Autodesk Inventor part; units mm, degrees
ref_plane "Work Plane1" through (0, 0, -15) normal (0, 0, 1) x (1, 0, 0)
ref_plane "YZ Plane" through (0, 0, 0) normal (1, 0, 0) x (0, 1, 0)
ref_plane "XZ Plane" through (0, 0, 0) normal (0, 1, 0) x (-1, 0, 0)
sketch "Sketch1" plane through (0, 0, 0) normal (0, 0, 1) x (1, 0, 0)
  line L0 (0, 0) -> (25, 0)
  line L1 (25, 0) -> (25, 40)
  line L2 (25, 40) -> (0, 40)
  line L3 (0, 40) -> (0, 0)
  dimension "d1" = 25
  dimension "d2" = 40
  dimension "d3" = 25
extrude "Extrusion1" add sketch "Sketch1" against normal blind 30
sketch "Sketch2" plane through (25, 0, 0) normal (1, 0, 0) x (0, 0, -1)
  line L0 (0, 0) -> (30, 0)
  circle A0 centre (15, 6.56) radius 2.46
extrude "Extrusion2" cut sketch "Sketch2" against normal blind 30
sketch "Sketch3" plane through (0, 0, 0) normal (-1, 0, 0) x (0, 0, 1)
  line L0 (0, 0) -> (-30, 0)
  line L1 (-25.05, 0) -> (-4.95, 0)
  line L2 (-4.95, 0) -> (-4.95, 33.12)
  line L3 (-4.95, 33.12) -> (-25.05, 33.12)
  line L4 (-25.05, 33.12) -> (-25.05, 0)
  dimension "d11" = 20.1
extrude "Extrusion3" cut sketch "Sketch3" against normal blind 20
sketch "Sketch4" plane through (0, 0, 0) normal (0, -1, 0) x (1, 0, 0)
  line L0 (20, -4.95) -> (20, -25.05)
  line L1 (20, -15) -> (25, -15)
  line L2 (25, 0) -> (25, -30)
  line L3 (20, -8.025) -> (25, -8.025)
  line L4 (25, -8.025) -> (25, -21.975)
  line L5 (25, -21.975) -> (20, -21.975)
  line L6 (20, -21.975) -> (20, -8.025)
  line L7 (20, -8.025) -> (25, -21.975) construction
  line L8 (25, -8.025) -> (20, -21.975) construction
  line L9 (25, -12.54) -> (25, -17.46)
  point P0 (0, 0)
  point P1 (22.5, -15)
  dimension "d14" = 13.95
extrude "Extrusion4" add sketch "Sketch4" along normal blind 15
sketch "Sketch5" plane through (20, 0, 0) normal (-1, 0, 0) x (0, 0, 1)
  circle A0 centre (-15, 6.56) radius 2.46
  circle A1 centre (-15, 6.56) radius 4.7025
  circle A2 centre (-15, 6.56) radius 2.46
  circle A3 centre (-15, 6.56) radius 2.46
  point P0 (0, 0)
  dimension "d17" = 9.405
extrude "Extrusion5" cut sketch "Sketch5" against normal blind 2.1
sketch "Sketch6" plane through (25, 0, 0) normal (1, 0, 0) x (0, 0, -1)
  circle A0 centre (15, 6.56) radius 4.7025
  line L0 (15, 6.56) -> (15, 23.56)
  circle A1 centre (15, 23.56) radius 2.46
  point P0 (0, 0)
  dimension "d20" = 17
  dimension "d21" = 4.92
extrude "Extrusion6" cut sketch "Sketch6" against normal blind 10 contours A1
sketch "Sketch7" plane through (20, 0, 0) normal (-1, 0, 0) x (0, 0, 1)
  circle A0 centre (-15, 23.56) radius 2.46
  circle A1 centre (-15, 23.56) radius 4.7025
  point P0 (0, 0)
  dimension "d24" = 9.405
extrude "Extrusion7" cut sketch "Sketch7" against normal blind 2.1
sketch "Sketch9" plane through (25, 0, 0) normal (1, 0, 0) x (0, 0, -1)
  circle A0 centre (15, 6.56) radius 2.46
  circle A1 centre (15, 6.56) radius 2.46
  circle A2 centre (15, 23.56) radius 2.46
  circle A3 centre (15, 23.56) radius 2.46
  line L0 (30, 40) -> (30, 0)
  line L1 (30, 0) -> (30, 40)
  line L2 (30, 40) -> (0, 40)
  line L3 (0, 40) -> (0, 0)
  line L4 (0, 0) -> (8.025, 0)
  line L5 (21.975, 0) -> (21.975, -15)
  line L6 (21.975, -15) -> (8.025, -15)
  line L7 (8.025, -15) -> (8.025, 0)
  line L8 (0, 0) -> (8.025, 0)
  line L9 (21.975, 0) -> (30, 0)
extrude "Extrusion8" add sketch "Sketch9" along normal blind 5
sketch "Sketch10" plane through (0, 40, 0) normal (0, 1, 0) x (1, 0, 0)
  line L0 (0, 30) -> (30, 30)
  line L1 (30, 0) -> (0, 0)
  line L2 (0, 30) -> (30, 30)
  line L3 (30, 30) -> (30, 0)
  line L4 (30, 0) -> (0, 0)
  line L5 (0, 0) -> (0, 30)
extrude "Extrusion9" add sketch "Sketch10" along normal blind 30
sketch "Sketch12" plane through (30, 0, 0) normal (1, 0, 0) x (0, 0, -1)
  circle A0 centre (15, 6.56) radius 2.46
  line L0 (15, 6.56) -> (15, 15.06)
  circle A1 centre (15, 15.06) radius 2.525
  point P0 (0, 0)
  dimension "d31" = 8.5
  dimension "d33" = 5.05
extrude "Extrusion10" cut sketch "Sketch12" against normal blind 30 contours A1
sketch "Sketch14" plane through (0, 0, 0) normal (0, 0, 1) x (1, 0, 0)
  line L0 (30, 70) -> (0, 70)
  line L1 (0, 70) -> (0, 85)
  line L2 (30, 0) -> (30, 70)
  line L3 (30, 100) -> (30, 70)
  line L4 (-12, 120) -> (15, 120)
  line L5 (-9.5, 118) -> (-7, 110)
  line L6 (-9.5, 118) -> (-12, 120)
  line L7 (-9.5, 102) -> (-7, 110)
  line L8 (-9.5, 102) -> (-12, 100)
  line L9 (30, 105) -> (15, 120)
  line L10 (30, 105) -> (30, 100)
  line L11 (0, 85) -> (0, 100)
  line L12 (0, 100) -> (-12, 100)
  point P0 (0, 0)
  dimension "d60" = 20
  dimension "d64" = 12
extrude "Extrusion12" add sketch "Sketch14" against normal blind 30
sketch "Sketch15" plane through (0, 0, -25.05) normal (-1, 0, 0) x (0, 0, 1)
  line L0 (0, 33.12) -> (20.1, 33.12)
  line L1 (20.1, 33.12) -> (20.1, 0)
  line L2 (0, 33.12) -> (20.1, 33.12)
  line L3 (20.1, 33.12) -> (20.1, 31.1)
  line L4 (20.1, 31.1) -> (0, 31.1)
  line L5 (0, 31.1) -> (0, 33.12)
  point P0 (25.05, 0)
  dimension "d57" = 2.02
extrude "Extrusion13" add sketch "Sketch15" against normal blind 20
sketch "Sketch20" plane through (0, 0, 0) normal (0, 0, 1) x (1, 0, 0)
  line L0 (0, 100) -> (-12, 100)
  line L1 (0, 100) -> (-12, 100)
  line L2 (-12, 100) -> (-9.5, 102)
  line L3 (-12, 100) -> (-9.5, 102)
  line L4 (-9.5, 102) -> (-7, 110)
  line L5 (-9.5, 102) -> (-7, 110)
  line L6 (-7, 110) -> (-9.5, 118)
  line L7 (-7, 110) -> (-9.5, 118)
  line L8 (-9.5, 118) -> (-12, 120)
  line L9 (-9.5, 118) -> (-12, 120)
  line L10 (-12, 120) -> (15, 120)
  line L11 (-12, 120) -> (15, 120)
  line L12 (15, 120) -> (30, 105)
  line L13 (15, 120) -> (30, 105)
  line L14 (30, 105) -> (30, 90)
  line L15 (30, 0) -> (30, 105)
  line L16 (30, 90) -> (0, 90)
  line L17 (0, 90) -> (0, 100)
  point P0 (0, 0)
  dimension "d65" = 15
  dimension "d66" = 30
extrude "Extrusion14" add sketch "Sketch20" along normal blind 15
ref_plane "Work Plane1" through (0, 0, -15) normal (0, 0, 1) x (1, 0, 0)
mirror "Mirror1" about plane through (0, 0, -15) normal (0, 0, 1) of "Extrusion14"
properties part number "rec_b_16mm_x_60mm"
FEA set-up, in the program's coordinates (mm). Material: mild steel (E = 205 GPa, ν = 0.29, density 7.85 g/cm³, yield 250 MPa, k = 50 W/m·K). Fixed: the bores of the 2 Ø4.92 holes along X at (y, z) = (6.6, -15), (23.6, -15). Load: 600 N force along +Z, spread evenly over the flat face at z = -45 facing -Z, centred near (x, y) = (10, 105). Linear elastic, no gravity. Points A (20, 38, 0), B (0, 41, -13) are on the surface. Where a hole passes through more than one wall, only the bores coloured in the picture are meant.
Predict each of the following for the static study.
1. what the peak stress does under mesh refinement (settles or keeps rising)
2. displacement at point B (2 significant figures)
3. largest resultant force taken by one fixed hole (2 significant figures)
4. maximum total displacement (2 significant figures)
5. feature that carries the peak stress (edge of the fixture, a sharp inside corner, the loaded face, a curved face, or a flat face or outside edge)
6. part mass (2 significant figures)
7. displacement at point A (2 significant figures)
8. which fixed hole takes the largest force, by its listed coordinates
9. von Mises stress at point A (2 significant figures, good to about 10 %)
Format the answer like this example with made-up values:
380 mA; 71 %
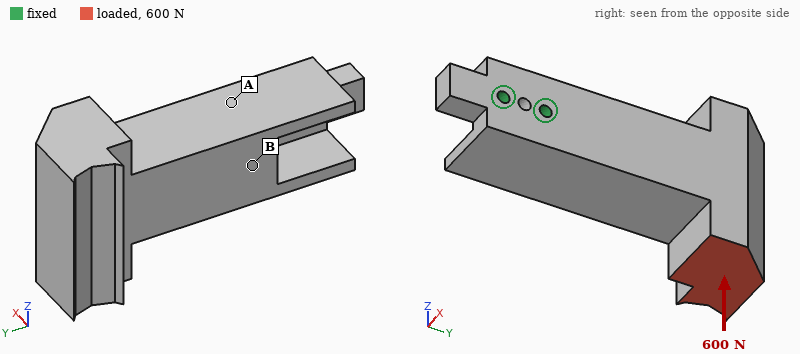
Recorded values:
keeps rising; 6.2 µm; 2.7 kN; 36 µm; edge of the fixture; 1.0 kg; 5.7 µm; (23.6, -15); 12 MPa
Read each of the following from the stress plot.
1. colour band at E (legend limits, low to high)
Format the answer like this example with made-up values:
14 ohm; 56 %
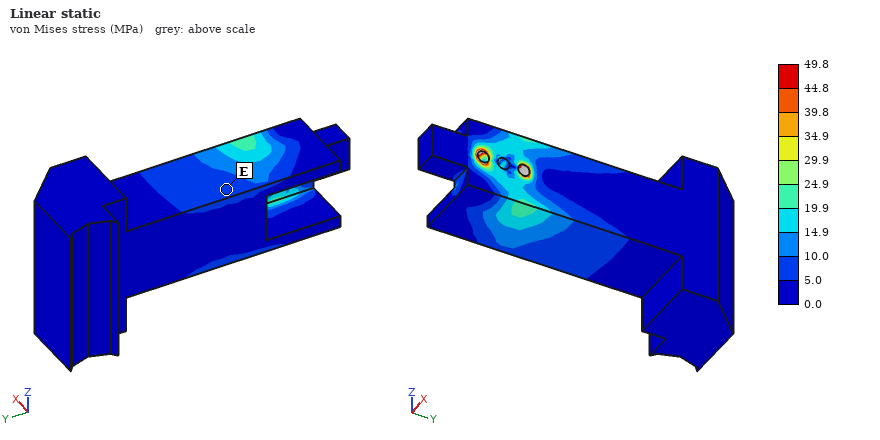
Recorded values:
5.0 to 10.0 MPa
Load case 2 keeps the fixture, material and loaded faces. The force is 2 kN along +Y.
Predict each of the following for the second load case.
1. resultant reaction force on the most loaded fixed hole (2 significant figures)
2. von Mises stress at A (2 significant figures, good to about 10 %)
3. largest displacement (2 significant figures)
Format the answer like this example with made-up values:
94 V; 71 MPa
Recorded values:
3.1 kN; 18 MPa; 59 µm
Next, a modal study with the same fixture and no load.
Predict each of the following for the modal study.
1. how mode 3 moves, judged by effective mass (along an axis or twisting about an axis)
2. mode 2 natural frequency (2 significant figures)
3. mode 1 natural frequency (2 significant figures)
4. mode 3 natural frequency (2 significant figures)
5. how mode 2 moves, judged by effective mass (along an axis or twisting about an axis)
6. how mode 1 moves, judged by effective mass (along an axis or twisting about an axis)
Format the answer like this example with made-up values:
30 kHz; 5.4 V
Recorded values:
twisting about Y; 990 Hz; 850 Hz; 2200 Hz; along Z; along X
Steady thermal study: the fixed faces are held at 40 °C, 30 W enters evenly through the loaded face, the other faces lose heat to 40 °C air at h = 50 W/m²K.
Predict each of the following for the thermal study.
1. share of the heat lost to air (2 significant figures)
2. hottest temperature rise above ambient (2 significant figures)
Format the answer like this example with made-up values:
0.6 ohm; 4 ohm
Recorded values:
66 %; 44 K
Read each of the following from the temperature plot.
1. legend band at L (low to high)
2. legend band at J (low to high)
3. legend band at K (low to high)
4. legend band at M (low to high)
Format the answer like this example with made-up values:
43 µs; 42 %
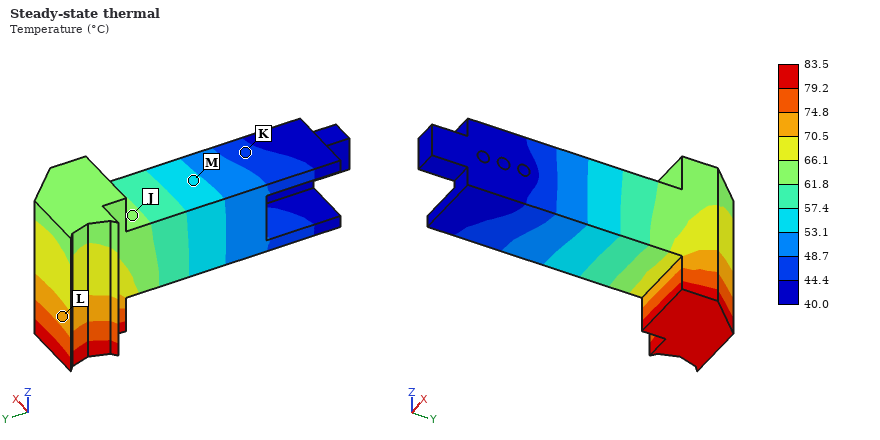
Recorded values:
70.5 to 74.8 °C; 61.8 to 66.1 °C; 44.4 to 48.7 °C; 53.1 to 57.4 °C
